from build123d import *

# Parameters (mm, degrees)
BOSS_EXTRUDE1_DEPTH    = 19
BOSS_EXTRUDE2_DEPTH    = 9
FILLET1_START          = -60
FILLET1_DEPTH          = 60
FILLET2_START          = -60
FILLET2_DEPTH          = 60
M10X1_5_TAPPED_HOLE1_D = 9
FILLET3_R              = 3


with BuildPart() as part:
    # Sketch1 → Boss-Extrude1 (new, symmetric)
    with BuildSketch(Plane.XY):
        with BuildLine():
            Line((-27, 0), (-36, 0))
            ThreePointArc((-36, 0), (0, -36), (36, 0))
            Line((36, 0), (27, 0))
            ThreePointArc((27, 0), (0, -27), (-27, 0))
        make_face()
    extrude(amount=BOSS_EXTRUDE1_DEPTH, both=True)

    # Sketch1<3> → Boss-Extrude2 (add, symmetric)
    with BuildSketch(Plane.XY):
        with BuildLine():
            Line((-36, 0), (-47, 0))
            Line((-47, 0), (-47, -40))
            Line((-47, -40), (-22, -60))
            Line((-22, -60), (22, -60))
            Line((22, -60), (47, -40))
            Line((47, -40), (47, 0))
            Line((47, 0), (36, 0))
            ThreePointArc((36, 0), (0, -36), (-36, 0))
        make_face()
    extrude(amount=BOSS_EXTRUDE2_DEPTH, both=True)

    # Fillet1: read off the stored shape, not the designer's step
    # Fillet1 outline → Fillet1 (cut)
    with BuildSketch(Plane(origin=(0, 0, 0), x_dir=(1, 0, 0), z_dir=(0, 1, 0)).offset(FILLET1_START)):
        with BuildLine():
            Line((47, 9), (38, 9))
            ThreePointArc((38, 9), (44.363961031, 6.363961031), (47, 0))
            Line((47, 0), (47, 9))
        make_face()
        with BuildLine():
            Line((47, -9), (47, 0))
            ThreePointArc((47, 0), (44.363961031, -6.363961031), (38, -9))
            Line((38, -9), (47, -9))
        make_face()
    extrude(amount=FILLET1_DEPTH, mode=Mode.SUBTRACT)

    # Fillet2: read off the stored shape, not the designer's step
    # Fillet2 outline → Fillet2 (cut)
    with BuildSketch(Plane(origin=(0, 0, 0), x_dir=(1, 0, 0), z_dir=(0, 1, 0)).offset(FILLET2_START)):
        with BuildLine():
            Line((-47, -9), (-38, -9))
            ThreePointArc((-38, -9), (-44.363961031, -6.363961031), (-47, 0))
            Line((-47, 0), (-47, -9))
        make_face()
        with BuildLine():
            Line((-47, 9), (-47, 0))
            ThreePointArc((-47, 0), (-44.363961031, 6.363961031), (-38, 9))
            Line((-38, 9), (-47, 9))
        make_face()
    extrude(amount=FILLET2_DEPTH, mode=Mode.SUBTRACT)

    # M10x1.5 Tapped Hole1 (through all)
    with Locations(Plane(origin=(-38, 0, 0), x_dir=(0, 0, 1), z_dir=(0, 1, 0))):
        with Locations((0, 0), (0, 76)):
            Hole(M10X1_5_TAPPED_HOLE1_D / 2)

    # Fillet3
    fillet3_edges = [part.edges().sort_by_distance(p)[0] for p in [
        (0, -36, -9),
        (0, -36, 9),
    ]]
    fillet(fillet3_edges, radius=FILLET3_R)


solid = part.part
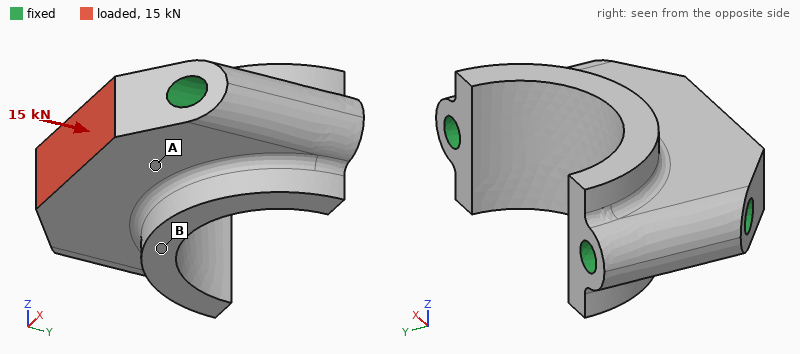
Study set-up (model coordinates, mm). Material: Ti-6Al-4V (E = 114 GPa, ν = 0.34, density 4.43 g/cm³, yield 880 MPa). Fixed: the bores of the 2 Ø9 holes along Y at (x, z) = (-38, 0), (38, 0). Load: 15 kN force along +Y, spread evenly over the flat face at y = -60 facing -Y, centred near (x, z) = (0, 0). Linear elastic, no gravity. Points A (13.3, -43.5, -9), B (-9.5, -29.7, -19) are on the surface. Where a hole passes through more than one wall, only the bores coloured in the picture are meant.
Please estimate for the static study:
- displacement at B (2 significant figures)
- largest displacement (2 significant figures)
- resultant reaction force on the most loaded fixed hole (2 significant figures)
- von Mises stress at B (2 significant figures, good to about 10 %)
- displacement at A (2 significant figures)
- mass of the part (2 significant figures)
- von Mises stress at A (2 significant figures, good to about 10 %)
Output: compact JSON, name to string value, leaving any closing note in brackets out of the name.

{"displacement at B": "4.9 µm", "largest displacement": "9.4 µm", "resultant reaction force on the most loaded fixed hole": "8.7 kN", "von Mises stress at B": "5.5 MPa", "displacement at A": "6.0 µm", "mass of the part": "360 g", "von Mises stress at A": "18 MPa"}
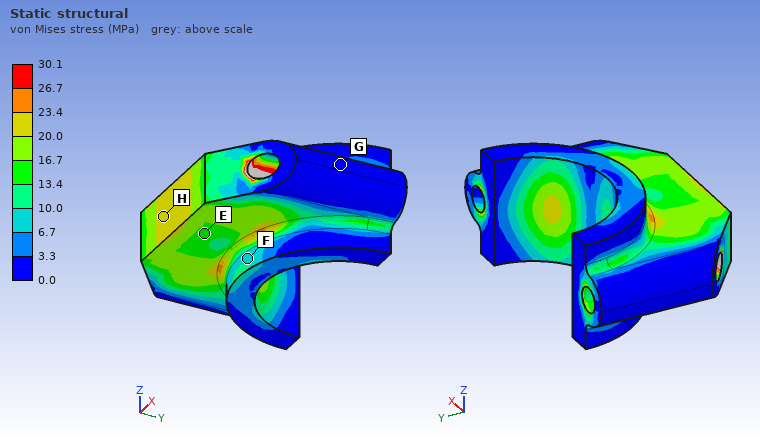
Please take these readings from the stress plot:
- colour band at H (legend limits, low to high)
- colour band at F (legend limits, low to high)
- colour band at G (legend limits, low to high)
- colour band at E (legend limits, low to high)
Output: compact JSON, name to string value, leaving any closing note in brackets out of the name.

{"colour band at H": "20.0 to 23.4 MPa", "colour band at F": "6.7 to 10.0 MPa", "colour band at G": "0.0 to 3.3 MPa", "colour band at E": "13.4 to 16.7 MPa"}
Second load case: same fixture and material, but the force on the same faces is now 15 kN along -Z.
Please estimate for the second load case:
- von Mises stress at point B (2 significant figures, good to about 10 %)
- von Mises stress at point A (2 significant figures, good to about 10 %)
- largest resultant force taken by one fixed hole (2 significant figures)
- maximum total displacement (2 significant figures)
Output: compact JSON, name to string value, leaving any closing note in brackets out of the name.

{"von Mises stress at point B": "24 MPa", "von Mises stress at point A": "71 MPa", "largest resultant force taken by one fixed hole": "7.5 kN", "maximum total displacement": "67 µm"}
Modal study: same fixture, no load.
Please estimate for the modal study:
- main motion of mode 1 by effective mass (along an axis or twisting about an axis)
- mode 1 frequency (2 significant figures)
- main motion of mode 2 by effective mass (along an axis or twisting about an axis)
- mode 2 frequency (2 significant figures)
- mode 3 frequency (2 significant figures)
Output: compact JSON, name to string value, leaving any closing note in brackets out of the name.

{"main motion of mode 1 by effective mass": "along Z", "mode 1 frequency": "12 kHz", "main motion of mode 2 by effective mass": "along Y", "mode 2 frequency": "19 kHz", "mode 3 frequency": "20 kHz"}
